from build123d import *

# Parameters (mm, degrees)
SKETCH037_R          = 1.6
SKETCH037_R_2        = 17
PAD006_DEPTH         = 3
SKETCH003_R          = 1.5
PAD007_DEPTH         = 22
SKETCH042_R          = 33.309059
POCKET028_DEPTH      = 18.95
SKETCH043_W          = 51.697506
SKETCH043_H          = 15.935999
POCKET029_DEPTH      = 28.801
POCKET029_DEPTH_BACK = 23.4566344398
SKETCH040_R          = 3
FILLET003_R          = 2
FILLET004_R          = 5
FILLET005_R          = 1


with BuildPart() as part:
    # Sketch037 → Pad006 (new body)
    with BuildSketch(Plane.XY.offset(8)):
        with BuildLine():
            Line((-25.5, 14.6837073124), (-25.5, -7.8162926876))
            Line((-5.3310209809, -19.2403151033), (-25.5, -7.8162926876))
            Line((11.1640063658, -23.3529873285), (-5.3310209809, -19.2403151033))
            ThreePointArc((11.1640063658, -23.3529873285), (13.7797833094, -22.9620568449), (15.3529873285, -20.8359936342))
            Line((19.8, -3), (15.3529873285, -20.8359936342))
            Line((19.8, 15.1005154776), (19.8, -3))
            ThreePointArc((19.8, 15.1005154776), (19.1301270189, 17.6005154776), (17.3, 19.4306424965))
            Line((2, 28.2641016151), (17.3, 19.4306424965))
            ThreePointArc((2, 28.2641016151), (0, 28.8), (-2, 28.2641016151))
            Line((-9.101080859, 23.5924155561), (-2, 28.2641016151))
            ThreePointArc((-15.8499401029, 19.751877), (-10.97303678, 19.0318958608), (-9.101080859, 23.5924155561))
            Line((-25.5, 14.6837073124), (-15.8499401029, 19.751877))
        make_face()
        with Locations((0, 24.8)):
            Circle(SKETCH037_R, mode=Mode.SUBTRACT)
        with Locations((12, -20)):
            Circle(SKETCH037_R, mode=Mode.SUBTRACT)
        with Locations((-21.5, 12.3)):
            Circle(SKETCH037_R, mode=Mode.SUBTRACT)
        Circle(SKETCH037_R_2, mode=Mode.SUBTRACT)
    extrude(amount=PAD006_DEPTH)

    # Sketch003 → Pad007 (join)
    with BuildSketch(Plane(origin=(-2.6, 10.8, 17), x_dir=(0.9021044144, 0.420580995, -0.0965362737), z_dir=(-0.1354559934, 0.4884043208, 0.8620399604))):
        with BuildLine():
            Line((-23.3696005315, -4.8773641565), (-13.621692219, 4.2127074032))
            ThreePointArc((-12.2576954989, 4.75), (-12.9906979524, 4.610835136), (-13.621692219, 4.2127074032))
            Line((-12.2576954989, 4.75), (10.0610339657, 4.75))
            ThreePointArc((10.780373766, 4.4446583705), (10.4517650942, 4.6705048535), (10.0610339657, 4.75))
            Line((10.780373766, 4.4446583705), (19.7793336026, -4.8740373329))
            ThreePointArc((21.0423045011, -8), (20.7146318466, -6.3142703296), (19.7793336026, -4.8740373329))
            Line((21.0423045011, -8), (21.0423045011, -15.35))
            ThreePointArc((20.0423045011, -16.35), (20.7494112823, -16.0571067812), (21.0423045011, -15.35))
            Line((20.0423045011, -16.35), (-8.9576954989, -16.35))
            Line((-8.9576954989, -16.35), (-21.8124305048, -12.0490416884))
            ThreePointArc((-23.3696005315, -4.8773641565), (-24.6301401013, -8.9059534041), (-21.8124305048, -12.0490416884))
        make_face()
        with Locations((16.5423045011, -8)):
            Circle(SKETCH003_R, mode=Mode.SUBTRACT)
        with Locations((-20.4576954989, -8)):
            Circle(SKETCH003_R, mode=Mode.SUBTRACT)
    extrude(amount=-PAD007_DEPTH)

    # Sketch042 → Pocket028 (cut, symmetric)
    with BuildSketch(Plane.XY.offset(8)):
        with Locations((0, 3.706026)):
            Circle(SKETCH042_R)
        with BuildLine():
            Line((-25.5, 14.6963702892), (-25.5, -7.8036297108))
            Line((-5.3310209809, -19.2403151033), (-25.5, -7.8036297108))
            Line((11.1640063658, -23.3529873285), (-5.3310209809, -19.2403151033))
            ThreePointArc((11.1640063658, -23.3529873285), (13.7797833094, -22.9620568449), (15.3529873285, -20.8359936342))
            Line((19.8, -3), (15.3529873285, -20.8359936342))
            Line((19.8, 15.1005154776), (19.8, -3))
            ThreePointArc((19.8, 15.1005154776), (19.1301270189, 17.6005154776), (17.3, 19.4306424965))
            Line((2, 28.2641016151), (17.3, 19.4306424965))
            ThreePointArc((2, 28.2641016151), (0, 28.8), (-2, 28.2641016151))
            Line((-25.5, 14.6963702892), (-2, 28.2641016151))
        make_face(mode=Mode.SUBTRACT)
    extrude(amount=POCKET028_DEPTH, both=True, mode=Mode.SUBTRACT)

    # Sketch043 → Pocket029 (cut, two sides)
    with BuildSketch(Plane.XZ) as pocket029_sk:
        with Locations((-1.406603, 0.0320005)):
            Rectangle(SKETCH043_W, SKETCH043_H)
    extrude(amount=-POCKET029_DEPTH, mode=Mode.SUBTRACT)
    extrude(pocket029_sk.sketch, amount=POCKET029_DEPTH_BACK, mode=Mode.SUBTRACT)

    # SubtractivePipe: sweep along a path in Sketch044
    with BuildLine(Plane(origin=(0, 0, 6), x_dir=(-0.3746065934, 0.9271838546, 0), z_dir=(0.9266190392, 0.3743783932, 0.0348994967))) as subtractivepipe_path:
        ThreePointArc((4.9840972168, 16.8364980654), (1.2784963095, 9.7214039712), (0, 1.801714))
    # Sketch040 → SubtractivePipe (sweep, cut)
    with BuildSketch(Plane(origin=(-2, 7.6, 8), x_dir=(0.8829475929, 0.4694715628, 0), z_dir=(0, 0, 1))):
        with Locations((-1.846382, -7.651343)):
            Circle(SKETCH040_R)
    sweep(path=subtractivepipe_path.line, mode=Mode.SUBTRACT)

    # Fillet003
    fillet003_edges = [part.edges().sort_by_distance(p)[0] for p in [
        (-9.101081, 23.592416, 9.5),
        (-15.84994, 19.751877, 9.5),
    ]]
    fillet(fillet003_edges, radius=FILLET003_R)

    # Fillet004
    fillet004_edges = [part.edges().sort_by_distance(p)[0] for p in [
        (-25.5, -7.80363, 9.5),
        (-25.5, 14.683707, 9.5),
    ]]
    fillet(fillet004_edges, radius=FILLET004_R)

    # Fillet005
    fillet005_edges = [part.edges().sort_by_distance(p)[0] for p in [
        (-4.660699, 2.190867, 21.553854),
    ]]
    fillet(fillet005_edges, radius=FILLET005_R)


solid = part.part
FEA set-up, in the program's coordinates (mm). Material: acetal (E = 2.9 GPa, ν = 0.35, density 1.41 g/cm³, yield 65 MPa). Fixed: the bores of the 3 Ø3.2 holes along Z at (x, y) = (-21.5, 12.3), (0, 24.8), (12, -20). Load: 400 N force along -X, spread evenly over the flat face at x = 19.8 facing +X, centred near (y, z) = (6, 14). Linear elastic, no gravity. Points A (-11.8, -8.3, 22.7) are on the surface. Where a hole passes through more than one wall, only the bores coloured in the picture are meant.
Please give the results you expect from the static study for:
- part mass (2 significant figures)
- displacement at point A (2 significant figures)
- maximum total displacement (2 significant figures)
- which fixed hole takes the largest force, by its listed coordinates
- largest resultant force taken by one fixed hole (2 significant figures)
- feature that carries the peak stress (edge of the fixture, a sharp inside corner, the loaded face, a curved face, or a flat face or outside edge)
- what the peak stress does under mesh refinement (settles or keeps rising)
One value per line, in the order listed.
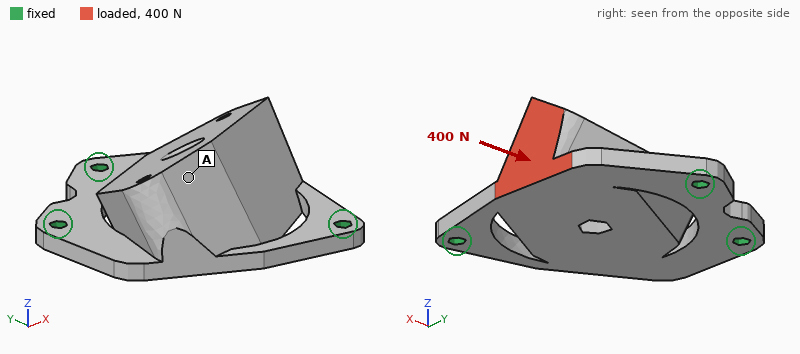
18 g
0.28 mm
0.44 mm
(0, 24.8)
190 N
edge of the fixture
keeps rising
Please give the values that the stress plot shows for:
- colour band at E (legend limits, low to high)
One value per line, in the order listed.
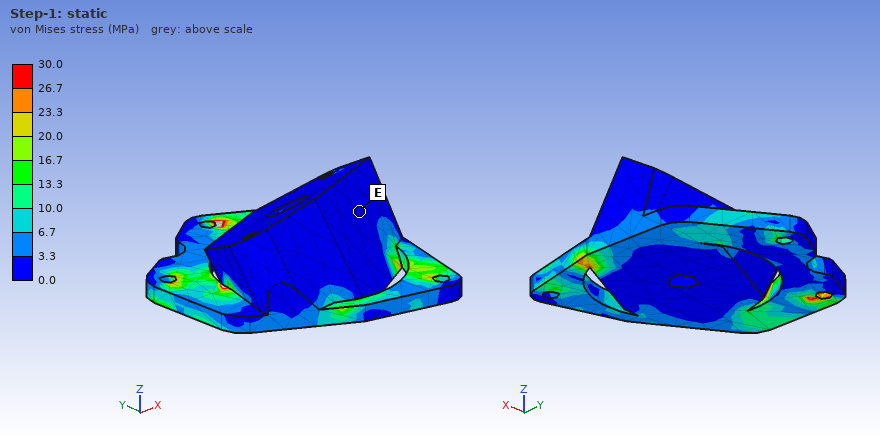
0.0 to 3.3 MPa
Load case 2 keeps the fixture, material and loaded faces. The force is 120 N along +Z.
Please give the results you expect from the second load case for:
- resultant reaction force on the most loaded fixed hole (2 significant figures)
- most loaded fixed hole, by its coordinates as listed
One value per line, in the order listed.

100 N
(0, 24.8)
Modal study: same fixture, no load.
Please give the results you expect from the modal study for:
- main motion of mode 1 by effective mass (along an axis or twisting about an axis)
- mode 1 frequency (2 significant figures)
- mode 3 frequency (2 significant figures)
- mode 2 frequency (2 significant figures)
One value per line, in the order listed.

along Z
850 Hz
2100 Hz
1100 Hz
